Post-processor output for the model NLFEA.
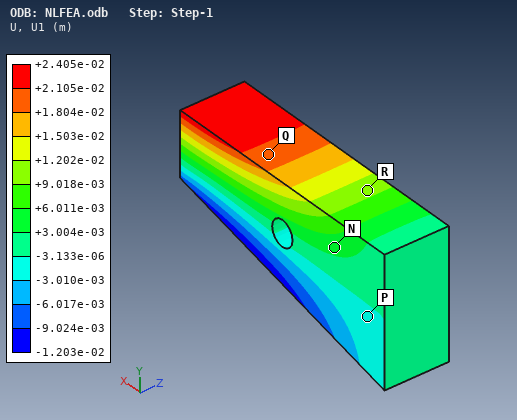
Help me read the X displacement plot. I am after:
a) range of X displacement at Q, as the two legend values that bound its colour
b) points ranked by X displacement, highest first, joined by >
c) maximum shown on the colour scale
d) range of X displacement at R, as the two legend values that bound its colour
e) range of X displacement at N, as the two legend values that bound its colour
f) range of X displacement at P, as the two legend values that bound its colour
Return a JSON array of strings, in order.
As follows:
["+1.804e-02 to +2.105e-02 m", "Q > R > N > P", "+2.405e-02 m", "+9.018e-03 to +1.202e-02 m", "+3.004e-03 to +6.011e-03 m", "-3.010e-03 to -3.133e-06 m"]
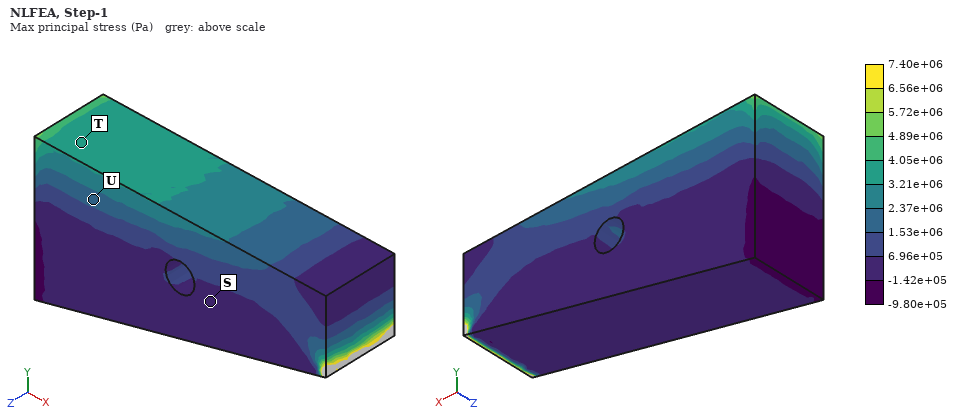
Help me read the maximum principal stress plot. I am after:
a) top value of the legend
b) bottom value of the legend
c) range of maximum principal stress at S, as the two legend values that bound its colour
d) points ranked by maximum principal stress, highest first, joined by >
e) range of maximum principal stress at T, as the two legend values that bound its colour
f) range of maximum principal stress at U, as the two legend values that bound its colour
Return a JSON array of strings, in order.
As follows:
["7.40e+06 Pa", "-9.80e+05 Pa", "-1.42e+05 to 6.96e+05 Pa", "T > U > S", "3.21e+06 to 4.05e+06 Pa", "1.53e+06 to 2.37e+06 Pa"]
